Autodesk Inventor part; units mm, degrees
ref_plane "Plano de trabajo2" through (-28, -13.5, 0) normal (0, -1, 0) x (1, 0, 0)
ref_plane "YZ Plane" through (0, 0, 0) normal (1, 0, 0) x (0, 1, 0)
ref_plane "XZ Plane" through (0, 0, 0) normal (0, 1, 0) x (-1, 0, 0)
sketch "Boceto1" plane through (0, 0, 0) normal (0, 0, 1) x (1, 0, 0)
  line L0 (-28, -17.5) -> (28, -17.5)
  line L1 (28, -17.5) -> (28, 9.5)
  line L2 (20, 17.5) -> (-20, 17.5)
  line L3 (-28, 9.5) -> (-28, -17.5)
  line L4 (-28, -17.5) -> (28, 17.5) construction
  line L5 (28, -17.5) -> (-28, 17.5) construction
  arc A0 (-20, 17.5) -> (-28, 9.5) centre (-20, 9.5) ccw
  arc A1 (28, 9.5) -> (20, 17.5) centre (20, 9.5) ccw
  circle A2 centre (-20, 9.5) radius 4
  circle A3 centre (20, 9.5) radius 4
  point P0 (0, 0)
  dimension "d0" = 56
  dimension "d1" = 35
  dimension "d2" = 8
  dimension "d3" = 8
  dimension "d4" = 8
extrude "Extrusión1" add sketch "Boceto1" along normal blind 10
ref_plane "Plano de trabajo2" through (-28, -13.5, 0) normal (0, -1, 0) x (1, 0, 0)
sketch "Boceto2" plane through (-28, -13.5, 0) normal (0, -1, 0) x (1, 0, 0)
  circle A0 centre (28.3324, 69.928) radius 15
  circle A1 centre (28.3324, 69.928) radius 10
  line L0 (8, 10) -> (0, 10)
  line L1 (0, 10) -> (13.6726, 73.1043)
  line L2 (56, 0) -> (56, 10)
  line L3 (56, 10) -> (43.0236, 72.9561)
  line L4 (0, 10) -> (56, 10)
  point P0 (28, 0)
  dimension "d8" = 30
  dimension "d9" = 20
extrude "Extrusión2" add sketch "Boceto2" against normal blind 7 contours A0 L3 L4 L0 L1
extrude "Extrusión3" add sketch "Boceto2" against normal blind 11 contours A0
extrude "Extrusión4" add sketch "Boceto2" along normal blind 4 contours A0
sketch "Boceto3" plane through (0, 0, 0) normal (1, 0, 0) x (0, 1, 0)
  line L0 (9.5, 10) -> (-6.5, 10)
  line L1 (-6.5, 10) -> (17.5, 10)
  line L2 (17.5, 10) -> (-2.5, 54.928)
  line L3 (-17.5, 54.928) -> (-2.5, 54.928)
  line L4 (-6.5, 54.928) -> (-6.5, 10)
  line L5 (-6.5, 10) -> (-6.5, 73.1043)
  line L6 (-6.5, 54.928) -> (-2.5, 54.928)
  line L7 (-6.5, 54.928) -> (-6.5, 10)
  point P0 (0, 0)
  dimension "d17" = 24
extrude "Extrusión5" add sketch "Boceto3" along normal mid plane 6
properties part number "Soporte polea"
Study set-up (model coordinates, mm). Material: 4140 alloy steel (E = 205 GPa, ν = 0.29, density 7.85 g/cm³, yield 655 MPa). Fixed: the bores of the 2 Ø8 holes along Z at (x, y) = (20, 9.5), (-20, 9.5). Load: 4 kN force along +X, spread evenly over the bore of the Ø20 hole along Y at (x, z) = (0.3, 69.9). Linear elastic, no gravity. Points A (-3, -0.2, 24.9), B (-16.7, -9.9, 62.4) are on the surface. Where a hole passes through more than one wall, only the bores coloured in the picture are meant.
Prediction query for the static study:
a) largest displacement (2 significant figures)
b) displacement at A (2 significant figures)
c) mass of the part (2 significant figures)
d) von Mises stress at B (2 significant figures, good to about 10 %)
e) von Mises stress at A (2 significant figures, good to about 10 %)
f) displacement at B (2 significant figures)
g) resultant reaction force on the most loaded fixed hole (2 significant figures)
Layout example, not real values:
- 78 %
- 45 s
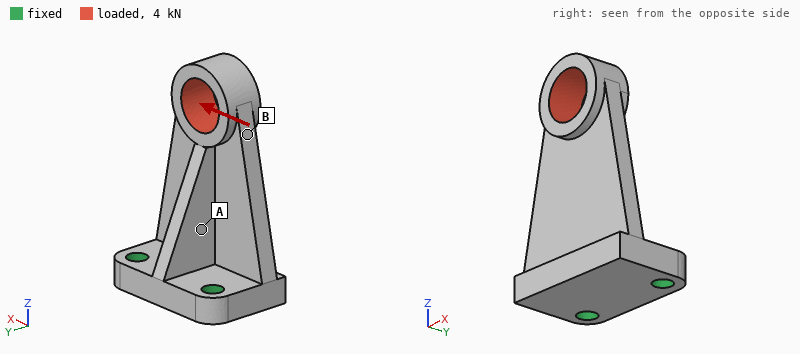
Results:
- 0.13 mm
- 0.024 mm
- 340 g
- 78 MPa
- 31 MPa
- 0.088 mm
- 6.8 kN
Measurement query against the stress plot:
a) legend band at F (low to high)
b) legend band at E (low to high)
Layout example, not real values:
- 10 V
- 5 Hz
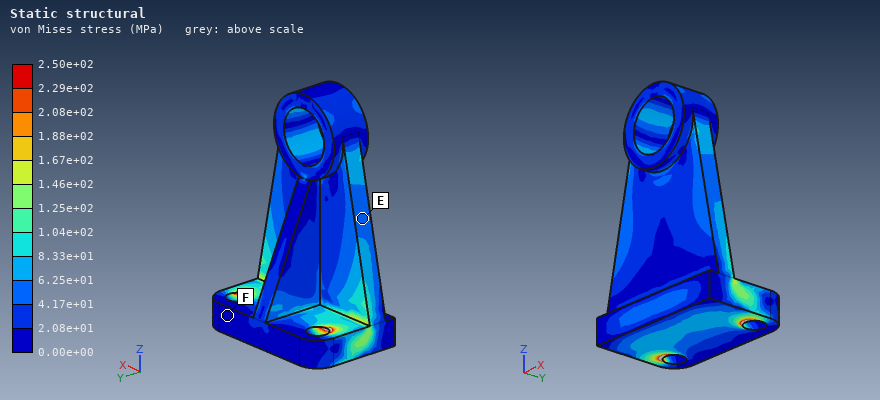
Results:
- 0.00e+00 to 2.08e+01 MPa
- 4.17e+01 to 6.25e+01 MPa
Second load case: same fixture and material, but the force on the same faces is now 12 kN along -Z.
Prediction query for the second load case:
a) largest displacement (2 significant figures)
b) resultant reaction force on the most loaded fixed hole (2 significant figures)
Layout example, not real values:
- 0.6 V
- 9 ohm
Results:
- 0.18 mm
- 6.1 kN
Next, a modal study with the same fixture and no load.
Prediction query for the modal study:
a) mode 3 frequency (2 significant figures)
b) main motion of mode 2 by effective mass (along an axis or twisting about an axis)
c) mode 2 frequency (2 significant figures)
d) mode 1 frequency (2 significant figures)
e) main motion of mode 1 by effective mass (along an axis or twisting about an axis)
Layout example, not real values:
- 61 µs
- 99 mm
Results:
- 5200 Hz
- along X
- 3500 Hz
- 2000 Hz
- along Y
